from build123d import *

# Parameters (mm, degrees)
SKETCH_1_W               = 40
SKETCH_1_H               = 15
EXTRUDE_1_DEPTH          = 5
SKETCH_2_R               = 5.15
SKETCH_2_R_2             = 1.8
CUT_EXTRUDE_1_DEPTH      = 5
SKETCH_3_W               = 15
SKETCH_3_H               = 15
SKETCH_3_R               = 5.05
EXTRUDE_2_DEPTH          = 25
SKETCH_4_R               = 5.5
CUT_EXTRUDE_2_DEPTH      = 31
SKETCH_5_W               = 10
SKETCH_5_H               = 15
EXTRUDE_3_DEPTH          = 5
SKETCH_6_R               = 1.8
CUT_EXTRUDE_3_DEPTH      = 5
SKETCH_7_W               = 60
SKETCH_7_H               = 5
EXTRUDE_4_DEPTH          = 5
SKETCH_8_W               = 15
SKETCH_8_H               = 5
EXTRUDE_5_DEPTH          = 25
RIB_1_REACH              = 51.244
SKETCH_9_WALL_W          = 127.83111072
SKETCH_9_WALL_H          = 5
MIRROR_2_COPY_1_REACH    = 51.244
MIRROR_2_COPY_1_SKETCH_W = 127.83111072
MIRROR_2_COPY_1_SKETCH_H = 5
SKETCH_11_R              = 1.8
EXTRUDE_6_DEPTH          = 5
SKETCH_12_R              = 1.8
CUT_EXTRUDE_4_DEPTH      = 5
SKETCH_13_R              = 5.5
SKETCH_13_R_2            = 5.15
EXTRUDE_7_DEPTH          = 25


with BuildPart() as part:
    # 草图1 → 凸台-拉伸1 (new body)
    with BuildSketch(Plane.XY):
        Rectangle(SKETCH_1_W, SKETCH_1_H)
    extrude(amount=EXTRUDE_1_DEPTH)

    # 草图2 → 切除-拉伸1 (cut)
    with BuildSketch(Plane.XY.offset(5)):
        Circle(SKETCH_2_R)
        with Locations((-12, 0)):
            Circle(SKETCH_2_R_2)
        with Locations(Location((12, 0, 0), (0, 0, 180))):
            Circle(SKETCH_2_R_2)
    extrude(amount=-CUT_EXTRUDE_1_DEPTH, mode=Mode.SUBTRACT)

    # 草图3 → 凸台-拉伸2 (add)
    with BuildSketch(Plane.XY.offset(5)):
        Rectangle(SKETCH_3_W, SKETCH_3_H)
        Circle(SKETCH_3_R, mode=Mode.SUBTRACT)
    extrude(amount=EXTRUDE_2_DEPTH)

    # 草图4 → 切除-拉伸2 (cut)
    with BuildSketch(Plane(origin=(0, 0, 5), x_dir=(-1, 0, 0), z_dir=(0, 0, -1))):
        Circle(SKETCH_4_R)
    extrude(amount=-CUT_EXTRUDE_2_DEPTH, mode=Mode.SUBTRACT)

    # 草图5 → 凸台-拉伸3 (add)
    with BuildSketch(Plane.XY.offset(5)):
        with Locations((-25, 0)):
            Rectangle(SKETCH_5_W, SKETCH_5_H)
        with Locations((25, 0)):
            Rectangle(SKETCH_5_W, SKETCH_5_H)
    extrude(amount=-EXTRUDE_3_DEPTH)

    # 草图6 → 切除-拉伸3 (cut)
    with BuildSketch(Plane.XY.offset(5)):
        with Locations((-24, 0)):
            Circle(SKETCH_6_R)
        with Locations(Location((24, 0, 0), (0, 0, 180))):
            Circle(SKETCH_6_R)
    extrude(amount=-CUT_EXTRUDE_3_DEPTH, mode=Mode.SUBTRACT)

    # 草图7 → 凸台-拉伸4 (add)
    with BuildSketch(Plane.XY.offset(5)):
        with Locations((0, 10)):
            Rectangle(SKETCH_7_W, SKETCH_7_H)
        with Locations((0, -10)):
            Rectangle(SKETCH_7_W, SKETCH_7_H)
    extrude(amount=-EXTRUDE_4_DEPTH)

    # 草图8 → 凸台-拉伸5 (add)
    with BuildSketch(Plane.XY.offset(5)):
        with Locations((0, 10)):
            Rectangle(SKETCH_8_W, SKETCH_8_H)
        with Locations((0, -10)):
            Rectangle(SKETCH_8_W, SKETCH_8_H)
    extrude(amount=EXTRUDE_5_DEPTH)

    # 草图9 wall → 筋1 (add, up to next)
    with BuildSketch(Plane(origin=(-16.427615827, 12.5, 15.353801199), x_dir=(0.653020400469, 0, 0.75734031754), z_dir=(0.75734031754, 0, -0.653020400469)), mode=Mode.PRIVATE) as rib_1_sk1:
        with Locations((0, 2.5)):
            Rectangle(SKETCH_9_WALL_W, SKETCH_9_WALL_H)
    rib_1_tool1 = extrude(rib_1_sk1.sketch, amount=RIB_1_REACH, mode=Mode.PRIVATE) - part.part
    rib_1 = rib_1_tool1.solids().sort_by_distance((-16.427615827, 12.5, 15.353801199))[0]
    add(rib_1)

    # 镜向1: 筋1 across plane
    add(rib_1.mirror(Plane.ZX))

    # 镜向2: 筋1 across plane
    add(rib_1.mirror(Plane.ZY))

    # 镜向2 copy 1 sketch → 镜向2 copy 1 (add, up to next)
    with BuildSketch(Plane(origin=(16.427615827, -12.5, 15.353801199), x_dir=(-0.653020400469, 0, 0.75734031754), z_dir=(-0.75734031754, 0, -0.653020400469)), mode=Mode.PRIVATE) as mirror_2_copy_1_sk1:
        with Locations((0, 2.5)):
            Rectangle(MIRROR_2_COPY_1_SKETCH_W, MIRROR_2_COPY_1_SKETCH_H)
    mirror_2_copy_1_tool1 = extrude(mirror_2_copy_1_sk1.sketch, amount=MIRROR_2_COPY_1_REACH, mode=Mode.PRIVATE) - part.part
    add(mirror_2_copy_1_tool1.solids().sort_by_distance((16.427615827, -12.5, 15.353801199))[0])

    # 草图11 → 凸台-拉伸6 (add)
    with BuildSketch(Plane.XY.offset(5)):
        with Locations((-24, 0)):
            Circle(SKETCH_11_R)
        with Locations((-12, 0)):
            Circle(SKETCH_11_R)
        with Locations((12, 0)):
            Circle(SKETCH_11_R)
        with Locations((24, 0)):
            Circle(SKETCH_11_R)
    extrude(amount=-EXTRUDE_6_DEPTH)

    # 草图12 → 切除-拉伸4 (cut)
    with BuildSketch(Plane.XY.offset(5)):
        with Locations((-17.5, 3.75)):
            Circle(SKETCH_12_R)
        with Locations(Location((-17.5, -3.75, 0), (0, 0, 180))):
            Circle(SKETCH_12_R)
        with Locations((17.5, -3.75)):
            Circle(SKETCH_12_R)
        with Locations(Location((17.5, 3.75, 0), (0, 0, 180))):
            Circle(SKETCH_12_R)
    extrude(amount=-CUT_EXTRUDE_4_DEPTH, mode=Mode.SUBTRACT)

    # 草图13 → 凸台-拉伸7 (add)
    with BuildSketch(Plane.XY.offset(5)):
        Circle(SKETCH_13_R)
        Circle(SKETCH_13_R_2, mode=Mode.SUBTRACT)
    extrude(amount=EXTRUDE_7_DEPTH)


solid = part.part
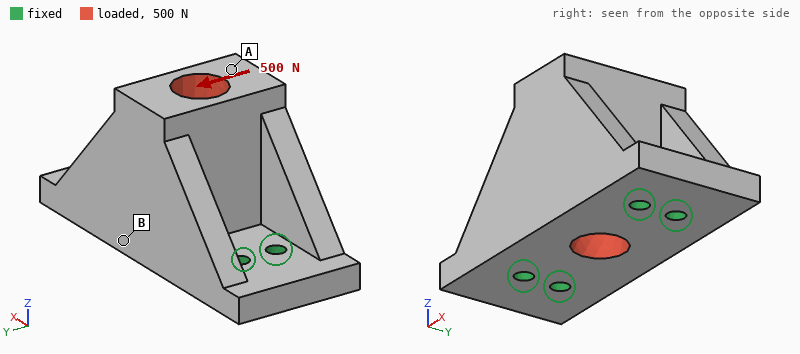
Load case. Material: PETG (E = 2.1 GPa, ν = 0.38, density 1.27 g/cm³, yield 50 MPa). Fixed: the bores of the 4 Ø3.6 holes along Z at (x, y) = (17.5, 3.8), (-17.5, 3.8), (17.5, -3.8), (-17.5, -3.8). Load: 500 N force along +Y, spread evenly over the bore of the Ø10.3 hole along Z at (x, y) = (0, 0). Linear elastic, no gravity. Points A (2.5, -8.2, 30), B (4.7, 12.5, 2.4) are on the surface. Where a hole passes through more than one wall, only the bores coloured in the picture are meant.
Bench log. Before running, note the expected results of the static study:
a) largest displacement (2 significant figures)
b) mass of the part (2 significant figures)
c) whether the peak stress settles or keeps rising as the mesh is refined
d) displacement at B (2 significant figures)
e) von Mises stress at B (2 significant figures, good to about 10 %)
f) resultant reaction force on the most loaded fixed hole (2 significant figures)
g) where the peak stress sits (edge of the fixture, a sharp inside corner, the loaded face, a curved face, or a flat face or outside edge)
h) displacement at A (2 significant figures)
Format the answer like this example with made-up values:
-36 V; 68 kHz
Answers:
0.35 mm; 23 g; keeps rising; 0.12 mm; 4.7 MPa; 270 N; edge of the fixture; 0.34 mm
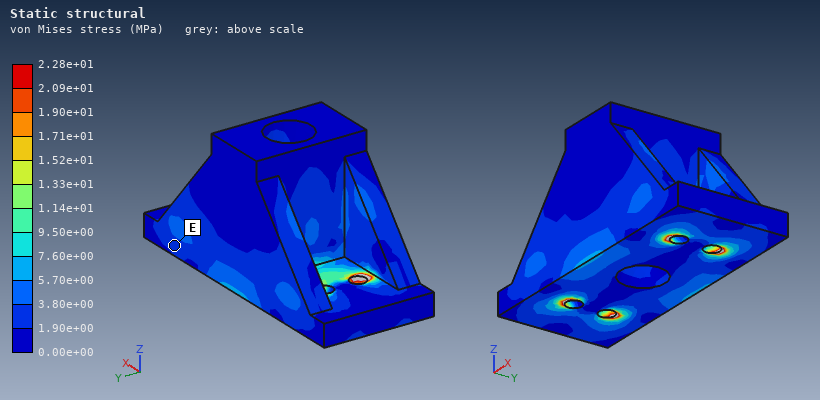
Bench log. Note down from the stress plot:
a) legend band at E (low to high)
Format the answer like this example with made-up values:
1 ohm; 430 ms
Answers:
1.90e+00 to 3.80e+00 MPa
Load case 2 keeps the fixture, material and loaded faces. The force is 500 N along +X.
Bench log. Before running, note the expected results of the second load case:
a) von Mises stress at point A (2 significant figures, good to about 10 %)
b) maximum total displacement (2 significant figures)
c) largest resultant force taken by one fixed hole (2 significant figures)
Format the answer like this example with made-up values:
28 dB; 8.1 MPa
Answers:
1.2 MPa; 75 µm; 150 N
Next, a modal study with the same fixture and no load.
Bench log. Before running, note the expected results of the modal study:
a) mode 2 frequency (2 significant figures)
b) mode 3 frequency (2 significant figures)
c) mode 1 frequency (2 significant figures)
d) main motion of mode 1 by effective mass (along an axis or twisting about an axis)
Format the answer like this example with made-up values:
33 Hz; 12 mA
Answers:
4200 Hz; 4300 Hz; 1800 Hz; along Y
